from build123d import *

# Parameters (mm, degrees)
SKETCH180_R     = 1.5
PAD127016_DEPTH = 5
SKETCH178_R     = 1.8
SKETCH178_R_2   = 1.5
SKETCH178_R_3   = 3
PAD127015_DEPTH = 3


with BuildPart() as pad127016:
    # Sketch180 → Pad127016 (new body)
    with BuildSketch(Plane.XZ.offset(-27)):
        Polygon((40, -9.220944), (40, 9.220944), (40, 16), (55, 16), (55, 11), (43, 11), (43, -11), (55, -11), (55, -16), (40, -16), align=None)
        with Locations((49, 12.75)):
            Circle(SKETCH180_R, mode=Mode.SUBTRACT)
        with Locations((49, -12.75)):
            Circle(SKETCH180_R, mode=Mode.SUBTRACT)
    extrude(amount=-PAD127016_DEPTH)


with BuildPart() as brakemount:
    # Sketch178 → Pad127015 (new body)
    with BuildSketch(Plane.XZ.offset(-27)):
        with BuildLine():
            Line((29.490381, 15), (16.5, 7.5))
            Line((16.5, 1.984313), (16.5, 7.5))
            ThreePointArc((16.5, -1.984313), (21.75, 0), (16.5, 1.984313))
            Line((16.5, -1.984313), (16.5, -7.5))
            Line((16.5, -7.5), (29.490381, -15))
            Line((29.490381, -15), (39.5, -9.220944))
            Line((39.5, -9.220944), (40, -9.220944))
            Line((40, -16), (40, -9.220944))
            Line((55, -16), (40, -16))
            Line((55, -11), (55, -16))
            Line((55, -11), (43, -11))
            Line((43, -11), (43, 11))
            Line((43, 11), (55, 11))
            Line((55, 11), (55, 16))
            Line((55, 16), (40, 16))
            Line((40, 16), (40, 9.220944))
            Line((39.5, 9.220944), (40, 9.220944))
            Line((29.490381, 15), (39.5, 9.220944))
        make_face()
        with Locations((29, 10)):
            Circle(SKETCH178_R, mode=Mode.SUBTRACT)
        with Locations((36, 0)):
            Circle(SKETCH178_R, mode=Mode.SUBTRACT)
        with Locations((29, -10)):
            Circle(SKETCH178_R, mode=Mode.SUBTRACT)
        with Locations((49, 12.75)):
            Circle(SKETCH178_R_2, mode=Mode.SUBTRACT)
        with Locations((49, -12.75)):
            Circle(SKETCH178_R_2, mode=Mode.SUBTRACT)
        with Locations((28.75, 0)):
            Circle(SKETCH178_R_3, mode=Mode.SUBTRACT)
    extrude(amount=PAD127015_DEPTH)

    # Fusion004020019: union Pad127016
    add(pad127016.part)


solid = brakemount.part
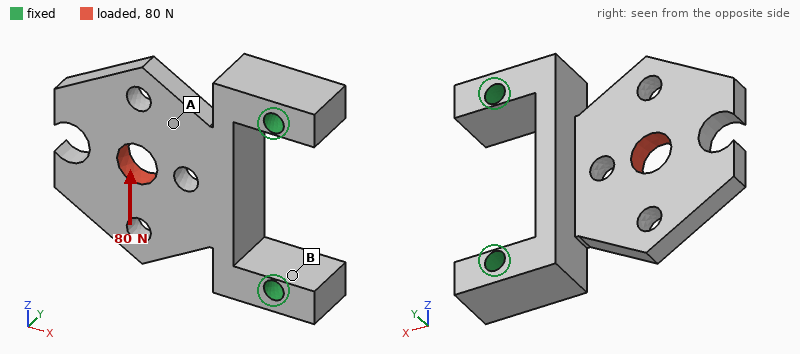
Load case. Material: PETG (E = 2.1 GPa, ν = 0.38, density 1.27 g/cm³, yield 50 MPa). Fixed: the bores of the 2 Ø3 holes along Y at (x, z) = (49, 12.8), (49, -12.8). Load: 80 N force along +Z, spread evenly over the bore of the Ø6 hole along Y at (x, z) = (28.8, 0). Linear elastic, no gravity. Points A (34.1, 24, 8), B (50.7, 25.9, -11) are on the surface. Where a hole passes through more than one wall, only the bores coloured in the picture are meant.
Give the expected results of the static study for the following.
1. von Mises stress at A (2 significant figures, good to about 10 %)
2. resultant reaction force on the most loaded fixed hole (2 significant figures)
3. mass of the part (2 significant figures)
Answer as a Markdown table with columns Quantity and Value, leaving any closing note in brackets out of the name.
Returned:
| Quantity | Value |
|---|---|
| von Mises stress at A | 2.0 MPa |
| resultant reaction force on the most loaded fixed hole | 65 N |
| mass of the part | 3.8 g |
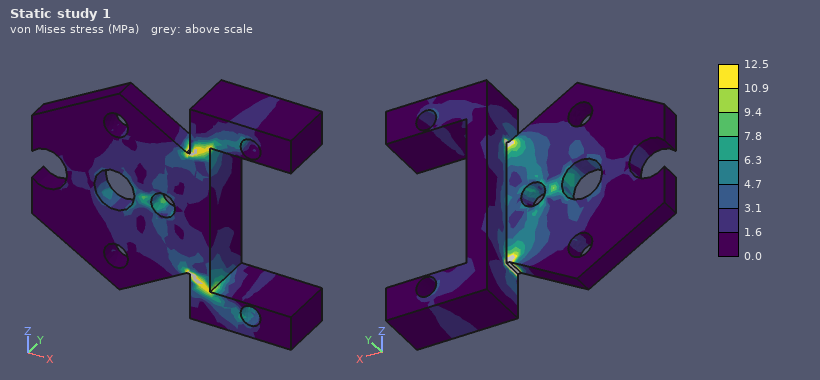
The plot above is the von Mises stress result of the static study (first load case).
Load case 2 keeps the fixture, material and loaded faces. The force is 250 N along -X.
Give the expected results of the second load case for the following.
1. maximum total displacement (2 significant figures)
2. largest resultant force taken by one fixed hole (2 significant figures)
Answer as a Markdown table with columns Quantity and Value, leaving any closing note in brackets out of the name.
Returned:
| Quantity | Value |
|---|---|
| maximum total displacement | 0.58 mm |
| largest resultant force taken by one fixed hole | 140 N |
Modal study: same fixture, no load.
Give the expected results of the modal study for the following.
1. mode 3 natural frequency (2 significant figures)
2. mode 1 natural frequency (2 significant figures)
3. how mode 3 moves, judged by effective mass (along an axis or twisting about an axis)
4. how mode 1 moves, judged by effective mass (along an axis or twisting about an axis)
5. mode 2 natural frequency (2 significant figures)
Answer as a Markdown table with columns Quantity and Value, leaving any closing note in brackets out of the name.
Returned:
| Quantity | Value |
|---|---|
| mode 3 natural frequency | 3000 Hz |
| mode 1 natural frequency | 780 Hz |
| how mode 3 moves, judged by effective mass | along Z |
| how mode 1 moves, judged by effective mass | along Y |
| mode 2 natural frequency | 2000 Hz |
